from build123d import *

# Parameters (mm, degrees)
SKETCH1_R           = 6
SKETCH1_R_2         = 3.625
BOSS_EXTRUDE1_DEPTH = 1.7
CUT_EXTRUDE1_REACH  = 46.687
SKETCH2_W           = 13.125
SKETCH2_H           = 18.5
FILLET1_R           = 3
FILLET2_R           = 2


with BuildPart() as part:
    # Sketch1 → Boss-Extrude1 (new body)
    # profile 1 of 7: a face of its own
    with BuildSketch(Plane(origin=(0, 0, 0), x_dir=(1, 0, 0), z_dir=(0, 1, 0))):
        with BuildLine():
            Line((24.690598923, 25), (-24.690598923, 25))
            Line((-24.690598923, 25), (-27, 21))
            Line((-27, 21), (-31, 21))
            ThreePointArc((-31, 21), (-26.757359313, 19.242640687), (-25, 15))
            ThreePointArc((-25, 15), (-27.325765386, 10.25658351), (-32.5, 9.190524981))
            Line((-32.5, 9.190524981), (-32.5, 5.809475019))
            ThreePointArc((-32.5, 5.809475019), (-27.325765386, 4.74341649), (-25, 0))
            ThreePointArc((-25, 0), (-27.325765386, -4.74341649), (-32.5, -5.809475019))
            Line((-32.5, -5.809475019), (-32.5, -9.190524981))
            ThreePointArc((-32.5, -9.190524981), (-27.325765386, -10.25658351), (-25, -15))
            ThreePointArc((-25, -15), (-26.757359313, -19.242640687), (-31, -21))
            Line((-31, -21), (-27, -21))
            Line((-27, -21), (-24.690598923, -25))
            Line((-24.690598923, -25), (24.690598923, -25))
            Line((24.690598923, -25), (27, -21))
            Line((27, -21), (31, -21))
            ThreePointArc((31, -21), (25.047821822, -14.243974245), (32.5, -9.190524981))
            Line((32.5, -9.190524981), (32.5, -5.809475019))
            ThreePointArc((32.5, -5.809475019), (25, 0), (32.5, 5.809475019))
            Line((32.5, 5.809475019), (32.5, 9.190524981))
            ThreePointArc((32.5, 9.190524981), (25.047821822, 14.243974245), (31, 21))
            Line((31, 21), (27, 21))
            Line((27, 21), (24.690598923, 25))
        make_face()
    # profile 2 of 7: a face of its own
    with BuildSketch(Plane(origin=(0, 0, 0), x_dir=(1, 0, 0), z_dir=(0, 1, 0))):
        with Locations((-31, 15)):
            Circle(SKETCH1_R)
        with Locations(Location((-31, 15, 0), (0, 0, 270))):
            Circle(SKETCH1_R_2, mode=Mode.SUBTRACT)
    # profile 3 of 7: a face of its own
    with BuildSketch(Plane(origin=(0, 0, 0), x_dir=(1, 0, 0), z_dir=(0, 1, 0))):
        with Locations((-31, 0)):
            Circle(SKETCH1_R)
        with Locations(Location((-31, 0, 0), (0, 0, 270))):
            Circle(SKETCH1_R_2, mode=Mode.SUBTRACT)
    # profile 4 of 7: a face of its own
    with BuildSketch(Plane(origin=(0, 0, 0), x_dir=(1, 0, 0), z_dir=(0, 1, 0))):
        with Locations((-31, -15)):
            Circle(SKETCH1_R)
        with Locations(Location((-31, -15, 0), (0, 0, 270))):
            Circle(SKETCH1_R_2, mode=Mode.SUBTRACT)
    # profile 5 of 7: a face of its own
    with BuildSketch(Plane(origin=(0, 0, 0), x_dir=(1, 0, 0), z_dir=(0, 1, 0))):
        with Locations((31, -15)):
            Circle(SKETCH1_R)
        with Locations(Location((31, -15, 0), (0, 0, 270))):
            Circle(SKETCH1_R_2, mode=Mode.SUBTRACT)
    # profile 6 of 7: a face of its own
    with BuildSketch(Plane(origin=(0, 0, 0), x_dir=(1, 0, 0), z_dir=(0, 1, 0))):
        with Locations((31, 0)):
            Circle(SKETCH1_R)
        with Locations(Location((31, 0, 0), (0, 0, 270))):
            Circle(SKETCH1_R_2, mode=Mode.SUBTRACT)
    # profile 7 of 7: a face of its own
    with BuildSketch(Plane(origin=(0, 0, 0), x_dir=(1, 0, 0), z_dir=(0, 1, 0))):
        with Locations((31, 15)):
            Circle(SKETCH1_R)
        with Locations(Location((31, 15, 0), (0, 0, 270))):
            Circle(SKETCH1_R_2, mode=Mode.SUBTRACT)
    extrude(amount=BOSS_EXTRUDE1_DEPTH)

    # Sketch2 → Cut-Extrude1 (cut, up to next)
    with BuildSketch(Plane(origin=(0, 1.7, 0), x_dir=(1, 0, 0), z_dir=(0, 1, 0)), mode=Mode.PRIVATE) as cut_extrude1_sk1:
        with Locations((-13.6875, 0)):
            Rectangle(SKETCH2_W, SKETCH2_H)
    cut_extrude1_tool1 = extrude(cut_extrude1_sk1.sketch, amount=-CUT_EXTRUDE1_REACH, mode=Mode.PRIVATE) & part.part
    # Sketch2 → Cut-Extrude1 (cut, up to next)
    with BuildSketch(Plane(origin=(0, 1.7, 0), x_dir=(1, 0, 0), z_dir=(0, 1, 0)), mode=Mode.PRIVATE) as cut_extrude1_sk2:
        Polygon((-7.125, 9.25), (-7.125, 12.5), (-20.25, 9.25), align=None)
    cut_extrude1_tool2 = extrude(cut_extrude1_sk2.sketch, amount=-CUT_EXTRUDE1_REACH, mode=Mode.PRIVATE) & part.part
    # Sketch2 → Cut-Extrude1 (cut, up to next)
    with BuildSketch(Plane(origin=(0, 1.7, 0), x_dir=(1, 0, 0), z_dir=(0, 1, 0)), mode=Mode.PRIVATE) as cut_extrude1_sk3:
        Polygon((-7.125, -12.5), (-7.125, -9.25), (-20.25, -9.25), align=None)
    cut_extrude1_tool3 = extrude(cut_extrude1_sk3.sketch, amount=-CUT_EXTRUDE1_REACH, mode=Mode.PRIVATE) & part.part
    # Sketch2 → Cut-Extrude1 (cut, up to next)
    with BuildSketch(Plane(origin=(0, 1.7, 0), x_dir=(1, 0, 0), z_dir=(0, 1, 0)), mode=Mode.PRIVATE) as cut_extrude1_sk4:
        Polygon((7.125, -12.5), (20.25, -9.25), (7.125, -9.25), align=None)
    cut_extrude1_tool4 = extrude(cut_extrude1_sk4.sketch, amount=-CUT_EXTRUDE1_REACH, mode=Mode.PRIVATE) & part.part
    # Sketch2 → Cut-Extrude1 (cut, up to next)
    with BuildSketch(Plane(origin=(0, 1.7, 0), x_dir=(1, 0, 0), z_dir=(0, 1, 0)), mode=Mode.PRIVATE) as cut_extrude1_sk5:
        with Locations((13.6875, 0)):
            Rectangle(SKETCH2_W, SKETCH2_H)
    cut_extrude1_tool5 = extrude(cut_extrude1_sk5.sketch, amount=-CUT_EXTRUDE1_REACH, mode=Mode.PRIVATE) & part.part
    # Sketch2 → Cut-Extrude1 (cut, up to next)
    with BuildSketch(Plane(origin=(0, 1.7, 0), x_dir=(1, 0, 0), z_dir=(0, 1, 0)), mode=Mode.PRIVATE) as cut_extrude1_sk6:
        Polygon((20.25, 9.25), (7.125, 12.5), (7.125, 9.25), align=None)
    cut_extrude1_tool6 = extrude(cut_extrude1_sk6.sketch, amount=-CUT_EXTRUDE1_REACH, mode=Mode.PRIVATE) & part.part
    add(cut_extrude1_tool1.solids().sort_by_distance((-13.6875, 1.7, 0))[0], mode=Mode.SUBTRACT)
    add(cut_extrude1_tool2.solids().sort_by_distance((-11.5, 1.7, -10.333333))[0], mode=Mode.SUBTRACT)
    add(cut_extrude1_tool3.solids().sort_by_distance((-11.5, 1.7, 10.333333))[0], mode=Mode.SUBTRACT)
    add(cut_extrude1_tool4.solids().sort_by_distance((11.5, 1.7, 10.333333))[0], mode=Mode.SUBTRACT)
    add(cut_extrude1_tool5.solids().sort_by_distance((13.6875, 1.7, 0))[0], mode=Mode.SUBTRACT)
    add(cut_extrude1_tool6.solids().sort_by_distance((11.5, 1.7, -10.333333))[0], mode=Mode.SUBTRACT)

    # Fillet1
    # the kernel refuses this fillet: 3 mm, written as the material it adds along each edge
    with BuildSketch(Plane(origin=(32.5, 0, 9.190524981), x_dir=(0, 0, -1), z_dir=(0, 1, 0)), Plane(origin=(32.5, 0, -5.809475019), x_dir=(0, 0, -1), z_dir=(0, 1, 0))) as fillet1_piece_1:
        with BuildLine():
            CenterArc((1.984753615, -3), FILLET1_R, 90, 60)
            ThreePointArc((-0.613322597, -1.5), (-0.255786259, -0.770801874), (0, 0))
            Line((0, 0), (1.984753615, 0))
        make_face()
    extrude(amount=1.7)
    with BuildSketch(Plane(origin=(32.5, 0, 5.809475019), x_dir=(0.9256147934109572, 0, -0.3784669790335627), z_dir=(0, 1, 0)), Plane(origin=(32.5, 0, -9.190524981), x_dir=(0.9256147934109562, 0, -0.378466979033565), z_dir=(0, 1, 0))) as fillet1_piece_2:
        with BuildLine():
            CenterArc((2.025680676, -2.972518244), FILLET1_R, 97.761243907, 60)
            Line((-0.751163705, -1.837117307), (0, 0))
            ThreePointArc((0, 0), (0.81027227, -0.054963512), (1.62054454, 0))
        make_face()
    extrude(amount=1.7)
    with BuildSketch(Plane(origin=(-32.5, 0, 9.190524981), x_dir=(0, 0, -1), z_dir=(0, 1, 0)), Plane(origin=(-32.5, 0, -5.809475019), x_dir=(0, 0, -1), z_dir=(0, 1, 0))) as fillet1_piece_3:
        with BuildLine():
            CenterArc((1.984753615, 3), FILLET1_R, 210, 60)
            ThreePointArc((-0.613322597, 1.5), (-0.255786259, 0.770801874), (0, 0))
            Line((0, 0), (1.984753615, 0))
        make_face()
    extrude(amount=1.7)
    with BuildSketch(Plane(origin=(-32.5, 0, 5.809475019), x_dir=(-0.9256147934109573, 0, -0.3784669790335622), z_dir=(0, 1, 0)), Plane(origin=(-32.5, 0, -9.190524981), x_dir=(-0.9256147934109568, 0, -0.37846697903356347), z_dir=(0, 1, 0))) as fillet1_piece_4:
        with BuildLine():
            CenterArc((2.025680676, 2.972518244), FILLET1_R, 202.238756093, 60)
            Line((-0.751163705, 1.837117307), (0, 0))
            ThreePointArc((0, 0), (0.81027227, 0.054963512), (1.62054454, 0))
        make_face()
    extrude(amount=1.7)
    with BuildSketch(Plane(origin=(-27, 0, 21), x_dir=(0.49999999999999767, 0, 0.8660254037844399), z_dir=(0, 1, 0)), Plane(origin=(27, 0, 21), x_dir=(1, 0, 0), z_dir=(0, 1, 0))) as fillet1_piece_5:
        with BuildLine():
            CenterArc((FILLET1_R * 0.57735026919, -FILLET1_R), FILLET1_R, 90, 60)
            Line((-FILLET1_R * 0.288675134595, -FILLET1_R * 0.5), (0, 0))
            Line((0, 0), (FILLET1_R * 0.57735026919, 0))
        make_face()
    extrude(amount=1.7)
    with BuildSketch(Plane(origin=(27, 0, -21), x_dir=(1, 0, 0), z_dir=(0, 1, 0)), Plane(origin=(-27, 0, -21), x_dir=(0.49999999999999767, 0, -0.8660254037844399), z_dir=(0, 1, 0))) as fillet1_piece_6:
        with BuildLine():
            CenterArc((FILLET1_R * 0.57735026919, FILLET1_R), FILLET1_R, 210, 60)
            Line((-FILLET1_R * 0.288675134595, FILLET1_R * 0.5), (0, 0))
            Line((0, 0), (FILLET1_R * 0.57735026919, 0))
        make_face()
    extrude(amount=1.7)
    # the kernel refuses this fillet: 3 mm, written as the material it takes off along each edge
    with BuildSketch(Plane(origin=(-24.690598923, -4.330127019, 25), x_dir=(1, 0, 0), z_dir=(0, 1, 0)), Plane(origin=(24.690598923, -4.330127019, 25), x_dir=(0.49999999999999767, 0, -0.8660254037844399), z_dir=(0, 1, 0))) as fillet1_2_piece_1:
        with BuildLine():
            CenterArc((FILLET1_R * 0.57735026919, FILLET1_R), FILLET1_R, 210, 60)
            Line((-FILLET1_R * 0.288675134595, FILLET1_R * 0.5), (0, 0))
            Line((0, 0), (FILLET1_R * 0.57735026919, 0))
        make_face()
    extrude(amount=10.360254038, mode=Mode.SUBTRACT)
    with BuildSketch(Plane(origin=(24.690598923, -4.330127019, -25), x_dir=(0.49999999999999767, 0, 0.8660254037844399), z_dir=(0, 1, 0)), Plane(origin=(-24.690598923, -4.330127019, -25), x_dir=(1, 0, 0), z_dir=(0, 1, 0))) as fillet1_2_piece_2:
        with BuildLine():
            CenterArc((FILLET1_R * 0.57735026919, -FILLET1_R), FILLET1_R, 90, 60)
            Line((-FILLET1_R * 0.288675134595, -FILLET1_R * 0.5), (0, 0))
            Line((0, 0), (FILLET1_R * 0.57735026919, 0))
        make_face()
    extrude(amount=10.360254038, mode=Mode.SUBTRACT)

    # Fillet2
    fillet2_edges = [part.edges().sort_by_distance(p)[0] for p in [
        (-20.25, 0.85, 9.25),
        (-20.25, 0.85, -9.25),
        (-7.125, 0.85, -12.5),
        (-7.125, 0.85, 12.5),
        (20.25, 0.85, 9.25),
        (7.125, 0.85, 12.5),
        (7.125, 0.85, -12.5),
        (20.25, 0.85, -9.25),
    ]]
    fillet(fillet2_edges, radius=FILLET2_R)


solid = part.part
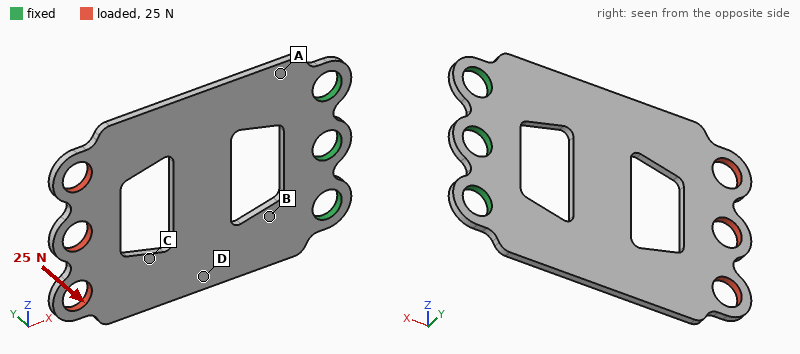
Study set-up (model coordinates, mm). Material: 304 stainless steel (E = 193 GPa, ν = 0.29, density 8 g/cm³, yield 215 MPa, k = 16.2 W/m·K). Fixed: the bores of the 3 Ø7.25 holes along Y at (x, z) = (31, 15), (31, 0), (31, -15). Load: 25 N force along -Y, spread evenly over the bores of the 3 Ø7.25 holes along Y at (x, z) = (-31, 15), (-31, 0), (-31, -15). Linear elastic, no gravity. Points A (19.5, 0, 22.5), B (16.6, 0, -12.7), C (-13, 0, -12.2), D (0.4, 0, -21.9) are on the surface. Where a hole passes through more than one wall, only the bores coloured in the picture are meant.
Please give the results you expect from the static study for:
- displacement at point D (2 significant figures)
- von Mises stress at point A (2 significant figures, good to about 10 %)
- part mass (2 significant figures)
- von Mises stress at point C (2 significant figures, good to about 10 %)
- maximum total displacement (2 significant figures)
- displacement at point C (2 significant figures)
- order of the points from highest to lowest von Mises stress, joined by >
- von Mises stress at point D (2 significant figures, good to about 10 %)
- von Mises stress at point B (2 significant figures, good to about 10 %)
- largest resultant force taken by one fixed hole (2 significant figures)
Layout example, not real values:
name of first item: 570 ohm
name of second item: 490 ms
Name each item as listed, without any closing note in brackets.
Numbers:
displacement at point D: 0.19 mm
von Mises stress at point A: 74 MPa
part mass: 35 g
von Mises stress at point C: 36 MPa
maximum total displacement: 0.81 mm
displacement at point C: 0.39 mm
order of the points from highest to lowest von Mises stress, joined by >: B > A > D > C
von Mises stress at point D: 50 MPa
von Mises stress at point B: 91 MPa
largest resultant force taken by one fixed hole: 14 N
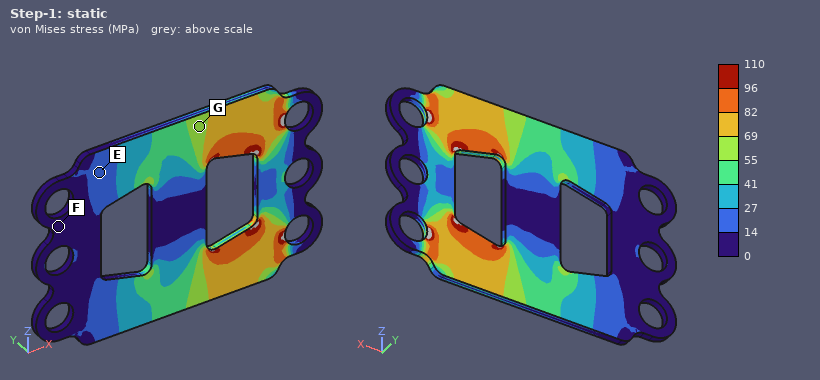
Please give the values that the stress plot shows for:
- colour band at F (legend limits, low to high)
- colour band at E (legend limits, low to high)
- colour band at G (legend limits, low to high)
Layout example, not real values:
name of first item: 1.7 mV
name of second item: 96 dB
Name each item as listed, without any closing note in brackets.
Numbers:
colour band at F: 0 to 14 MPa
colour band at E: 14 to 27 MPa
colour band at G: 55 to 69 MPa
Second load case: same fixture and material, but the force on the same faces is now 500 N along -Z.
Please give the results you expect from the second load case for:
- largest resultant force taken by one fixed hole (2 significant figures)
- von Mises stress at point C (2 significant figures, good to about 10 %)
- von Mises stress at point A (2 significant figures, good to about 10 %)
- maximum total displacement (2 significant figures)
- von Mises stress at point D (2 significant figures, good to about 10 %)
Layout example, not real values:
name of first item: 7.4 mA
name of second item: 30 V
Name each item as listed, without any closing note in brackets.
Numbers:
largest resultant force taken by one fixed hole: 830 N
von Mises stress at point C: 17 MPa
von Mises stress at point A: 43 MPa
maximum total displacement: 47 µm
von Mises stress at point D: 23 MPa
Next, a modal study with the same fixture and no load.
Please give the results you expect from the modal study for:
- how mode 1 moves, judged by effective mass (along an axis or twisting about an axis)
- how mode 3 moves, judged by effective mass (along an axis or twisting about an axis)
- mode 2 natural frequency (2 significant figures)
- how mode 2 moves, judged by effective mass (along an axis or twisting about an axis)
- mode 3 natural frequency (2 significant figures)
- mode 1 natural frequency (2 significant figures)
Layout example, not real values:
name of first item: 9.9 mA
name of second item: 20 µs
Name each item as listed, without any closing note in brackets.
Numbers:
how mode 1 moves, judged by effective mass: along Y
how mode 3 moves, judged by effective mass: along Y
mode 2 natural frequency: 960 Hz
how mode 2 moves, judged by effective mass: twisting about X
mode 3 natural frequency: 1900 Hz
mode 1 natural frequency: 320 Hz
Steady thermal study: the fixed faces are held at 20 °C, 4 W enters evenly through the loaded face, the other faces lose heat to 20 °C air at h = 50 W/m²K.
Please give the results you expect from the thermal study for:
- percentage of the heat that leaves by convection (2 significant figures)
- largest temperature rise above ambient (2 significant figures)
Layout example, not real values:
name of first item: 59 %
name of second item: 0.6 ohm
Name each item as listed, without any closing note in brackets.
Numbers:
percentage of the heat that leaves by convection: 98 %
largest temperature rise above ambient: 62 K
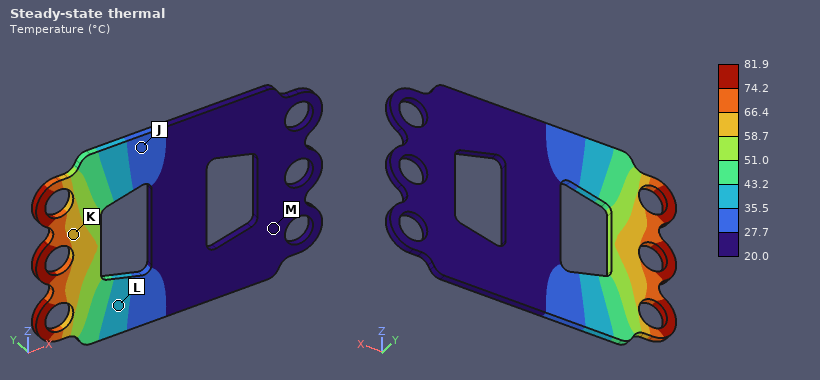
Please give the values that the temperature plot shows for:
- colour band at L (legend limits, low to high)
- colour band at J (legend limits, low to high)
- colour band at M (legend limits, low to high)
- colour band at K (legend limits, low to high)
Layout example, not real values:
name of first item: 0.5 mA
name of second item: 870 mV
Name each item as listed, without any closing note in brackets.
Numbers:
colour band at L: 35.5 to 43.2 °C
colour band at J: 27.7 to 35.5 °C
colour band at M: 20.0 to 27.7 °C
colour band at K: 58.7 to 66.4 °C
